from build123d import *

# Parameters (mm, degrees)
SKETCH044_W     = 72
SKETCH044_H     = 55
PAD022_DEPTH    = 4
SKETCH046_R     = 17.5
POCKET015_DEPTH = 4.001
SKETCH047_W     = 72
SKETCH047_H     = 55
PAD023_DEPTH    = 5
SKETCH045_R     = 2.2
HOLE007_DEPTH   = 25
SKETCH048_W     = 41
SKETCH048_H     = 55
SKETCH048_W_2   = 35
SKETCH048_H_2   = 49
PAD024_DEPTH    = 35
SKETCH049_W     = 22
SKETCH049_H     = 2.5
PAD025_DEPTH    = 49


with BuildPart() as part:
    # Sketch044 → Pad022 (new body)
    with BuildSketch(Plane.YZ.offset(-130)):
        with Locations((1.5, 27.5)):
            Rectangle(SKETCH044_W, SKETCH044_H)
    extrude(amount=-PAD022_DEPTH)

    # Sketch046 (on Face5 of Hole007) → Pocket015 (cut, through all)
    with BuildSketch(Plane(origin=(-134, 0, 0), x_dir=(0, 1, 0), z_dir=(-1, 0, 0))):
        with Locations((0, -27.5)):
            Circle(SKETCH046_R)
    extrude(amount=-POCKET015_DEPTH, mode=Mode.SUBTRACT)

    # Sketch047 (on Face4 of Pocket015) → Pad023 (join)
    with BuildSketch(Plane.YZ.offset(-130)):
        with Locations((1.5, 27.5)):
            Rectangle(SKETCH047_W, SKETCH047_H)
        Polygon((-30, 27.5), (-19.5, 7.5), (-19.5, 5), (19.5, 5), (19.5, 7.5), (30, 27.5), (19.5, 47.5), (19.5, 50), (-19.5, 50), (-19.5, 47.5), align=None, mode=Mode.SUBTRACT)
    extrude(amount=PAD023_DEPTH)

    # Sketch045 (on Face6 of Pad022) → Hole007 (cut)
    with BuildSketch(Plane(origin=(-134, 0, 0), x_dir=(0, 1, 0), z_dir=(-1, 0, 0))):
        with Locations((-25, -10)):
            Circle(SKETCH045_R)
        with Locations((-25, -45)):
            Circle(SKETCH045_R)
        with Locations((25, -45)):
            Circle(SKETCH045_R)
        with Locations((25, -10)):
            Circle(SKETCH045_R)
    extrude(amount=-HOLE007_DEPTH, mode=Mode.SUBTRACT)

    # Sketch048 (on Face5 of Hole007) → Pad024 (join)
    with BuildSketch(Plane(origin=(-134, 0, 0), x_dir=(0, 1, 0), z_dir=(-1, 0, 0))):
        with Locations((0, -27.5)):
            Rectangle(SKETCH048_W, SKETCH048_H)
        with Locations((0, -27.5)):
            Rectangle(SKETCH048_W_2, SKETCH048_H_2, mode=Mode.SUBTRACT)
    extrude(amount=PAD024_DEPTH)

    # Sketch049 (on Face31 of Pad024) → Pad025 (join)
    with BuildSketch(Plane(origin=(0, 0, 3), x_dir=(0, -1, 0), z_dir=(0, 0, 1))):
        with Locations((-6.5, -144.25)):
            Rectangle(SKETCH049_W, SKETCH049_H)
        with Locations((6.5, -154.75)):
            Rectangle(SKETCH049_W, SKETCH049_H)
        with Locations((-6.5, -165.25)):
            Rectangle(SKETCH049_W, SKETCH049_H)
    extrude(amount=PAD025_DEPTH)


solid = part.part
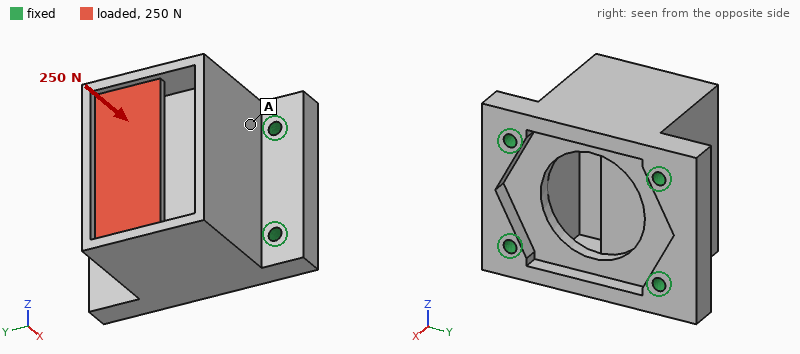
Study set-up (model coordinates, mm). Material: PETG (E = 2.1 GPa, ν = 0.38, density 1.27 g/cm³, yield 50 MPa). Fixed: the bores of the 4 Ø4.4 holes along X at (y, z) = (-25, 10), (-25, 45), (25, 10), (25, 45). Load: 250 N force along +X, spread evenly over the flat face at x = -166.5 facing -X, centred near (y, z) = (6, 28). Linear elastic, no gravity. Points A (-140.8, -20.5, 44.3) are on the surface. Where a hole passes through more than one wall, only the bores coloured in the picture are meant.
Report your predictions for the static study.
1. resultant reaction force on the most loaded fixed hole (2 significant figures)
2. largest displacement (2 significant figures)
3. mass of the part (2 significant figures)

84 N
1.1 mm
60 g
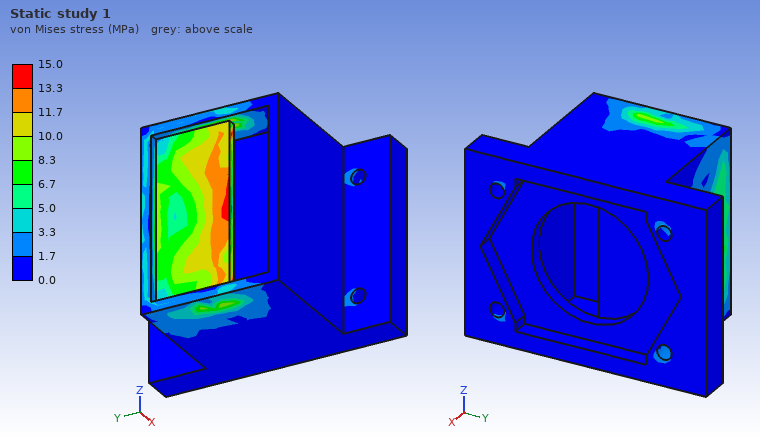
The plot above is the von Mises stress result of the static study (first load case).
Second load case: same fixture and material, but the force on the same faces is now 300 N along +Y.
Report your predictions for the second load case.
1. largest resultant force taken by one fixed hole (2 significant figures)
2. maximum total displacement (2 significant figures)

150 N
0.31 mm
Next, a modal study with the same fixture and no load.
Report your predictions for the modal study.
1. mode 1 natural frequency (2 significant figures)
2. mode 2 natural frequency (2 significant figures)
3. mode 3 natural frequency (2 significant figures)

1800 Hz
1800 Hz
1900 Hz
